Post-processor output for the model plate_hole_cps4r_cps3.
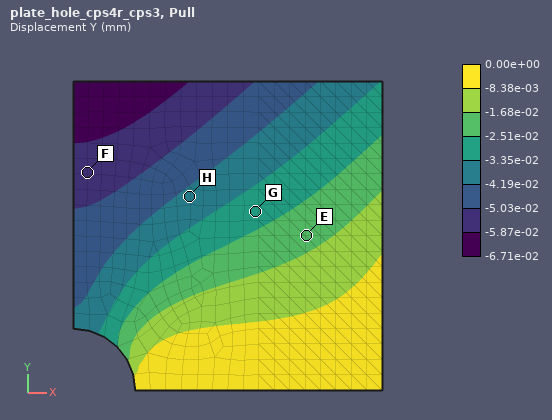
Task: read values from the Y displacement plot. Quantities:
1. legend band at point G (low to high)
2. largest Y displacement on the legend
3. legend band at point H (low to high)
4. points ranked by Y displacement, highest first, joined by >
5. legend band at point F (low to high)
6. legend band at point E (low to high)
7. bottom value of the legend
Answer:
-3.35e-02 to -2.51e-02 mm
0.00e+00 mm
-4.19e-02 to -3.35e-02 mm
E > G > H > F
-5.87e-02 to -5.03e-02 mm
-2.51e-02 to -1.68e-02 mm
-6.71e-02 mm
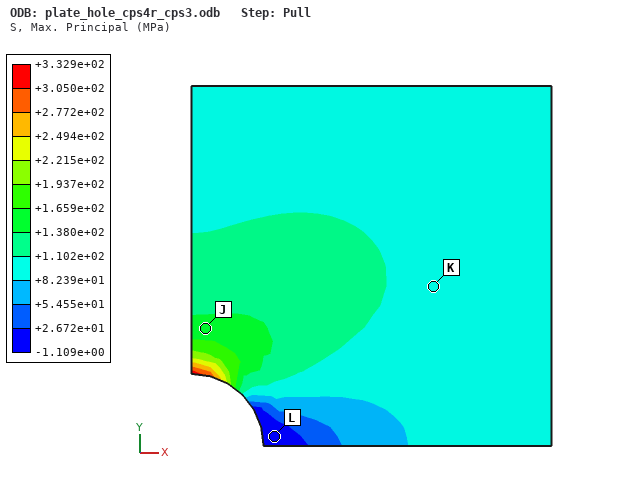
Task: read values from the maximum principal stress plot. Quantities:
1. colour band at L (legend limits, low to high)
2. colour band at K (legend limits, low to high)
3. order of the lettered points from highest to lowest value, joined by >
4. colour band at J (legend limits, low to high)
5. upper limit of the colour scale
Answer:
-1.109e+00 to +2.672e+01 MPa
+8.239e+01 to +1.102e+02 MPa
J > K > L
+1.380e+02 to +1.659e+02 MPa
+3.329e+02 MPa
